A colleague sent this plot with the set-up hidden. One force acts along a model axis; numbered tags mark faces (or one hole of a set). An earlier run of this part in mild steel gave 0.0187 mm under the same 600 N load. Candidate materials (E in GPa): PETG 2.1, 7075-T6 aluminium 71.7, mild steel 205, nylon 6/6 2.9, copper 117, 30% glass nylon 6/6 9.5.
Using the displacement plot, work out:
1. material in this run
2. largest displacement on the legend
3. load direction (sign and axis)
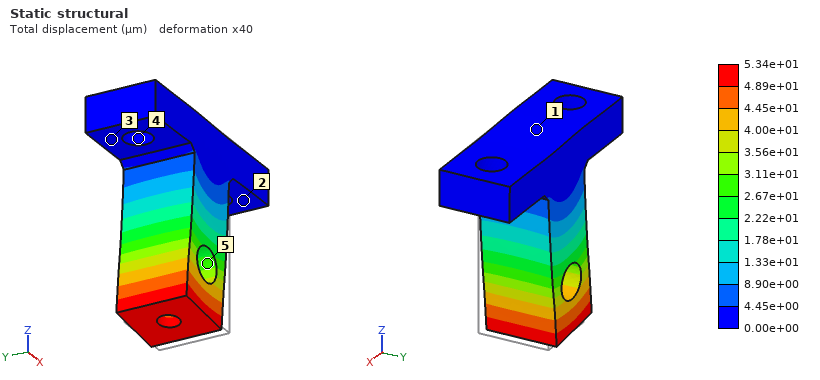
7075-T6 aluminium
5.34e+01 µm
-X
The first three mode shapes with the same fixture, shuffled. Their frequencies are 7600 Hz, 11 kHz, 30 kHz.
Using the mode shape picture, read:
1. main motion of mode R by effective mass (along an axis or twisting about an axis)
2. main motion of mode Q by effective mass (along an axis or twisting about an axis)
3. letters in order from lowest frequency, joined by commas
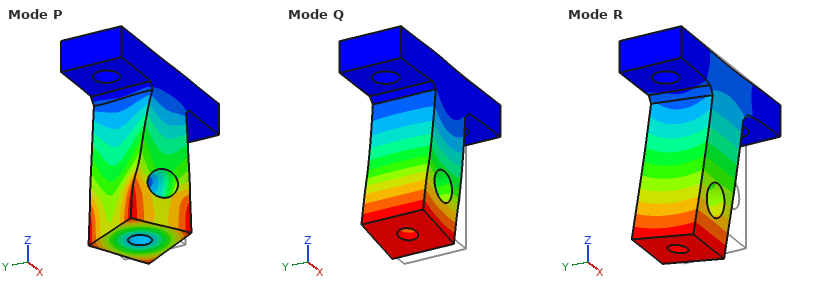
along Y
along X
R, Q, P
